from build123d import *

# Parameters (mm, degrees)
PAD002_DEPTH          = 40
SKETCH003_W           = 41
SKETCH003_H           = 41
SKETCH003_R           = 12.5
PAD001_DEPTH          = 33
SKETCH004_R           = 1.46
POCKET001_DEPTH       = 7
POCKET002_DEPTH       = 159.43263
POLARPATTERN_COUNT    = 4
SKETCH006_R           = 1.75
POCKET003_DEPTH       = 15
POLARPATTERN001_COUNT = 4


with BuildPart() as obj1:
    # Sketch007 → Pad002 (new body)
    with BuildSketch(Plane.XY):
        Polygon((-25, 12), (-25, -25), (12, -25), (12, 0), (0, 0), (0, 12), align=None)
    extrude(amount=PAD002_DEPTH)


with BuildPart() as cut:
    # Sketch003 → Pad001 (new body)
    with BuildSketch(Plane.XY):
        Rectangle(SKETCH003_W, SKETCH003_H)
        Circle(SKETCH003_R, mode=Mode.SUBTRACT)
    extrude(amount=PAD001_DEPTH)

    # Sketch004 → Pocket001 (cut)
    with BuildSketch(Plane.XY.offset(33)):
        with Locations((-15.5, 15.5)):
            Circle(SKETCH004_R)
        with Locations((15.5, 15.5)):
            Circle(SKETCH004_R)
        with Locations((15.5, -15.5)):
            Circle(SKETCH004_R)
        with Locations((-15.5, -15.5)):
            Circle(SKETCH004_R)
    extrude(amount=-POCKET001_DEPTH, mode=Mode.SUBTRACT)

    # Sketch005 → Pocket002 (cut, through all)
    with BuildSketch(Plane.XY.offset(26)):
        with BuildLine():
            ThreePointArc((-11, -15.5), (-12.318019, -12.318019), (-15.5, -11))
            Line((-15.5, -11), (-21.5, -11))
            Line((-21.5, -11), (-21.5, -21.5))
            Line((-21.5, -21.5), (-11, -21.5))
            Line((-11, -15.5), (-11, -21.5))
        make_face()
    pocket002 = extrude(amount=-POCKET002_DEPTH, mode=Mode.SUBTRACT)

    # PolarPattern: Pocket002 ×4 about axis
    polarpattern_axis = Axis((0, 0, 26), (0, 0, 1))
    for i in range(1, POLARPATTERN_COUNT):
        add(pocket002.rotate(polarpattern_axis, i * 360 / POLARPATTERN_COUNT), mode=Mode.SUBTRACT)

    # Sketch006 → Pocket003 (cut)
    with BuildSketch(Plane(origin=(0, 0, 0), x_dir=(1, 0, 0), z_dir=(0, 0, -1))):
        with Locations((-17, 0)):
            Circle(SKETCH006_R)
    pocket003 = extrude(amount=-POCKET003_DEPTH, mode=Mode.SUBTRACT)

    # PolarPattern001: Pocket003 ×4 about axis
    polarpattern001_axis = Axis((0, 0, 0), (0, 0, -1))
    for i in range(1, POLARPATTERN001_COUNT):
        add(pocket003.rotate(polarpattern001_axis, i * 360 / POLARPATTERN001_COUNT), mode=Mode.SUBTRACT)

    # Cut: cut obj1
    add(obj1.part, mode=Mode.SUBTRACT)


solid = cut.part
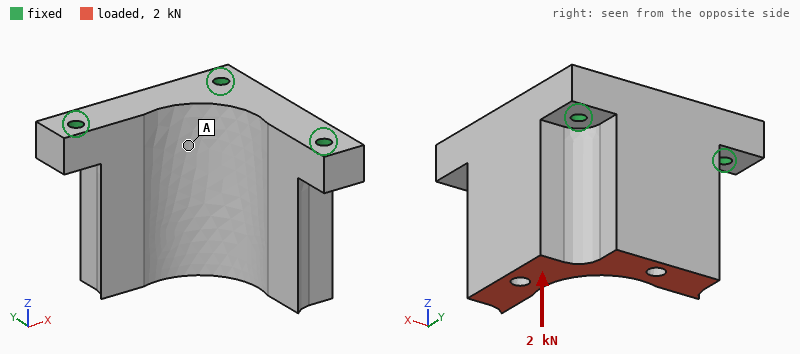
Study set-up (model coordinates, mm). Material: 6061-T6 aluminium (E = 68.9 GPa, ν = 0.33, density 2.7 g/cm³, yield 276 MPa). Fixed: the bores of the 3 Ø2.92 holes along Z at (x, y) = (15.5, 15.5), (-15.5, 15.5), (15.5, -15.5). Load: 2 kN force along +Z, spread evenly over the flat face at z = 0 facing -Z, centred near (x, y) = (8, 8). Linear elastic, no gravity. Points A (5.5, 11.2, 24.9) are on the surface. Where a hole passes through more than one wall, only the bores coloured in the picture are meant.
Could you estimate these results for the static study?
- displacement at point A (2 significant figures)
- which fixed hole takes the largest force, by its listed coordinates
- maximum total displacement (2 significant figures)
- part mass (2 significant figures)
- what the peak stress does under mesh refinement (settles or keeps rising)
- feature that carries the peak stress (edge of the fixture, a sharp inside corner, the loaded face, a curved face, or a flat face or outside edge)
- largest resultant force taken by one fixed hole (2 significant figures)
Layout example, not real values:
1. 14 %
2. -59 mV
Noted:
1. 3.7 µm
2. (15.5, 15.5)
3. 5.7 µm
4. 39 g
5. keeps rising
6. edge of the fixture
7. 1.1 kN
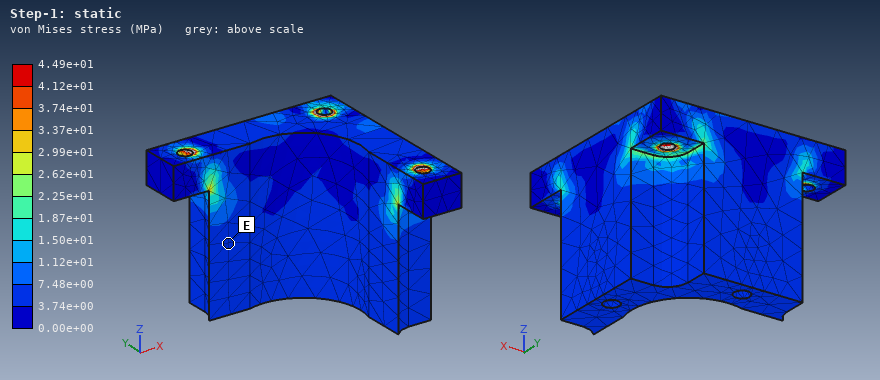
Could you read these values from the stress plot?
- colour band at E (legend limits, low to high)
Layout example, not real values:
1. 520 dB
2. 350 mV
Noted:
1. 3.74e+00 to 7.48e+00 MPa
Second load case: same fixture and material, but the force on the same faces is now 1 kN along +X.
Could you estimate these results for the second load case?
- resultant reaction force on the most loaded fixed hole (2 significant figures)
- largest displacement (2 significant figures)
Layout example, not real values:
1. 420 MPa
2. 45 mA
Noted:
1. 1.1 kN
2. 45 µm
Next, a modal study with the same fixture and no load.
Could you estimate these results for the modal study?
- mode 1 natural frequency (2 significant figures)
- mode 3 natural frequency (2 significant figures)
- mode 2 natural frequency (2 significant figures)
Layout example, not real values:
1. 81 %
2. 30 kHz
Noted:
1. 8100 Hz
2. 15 kHz
3. 9300 Hz
